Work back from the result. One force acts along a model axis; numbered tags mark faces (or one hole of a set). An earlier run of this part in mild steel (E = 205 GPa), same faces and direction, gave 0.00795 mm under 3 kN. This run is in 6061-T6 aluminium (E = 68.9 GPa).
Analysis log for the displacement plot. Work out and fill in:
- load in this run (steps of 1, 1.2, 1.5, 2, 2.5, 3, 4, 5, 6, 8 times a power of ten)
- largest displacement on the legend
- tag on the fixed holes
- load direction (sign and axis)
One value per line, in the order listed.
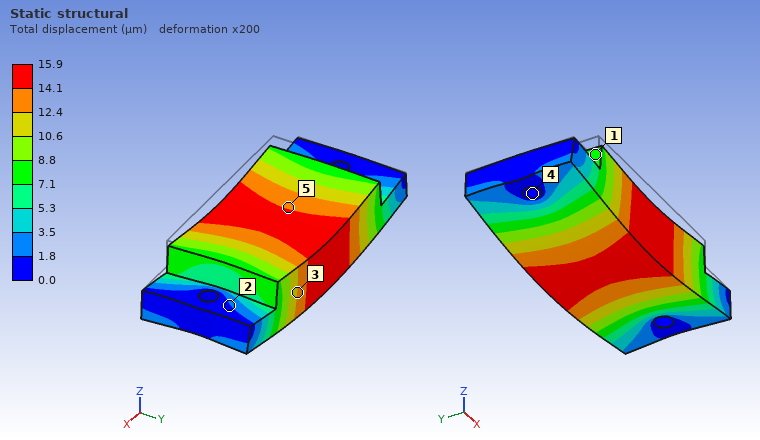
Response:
2 kN
15.9 µm
4
-Z
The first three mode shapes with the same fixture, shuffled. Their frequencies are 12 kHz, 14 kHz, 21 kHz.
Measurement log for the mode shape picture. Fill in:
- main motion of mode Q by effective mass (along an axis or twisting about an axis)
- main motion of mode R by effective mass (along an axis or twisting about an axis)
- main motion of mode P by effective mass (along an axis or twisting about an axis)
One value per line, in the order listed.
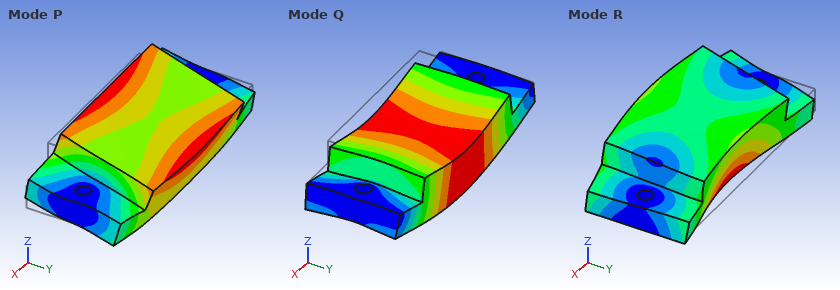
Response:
along Z
along Y
along Y
